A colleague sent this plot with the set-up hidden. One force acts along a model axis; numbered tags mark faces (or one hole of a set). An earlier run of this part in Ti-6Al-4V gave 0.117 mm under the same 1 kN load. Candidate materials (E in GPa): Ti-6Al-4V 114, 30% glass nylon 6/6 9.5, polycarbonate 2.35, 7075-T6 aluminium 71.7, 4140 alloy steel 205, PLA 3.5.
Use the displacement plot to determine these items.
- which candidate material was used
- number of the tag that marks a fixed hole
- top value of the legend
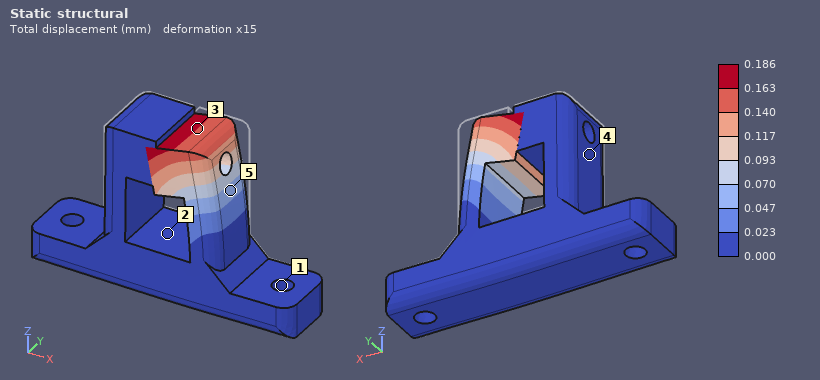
7075-T6 aluminium
1
0.186 mm
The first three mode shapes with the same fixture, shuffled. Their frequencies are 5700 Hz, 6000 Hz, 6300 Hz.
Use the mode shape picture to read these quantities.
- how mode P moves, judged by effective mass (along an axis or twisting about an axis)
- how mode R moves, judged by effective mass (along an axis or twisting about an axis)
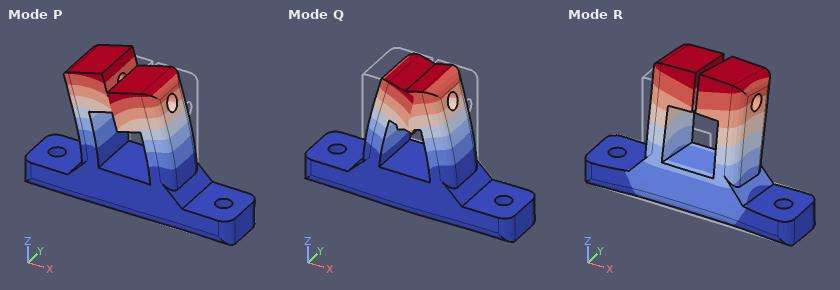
along X
along Y
